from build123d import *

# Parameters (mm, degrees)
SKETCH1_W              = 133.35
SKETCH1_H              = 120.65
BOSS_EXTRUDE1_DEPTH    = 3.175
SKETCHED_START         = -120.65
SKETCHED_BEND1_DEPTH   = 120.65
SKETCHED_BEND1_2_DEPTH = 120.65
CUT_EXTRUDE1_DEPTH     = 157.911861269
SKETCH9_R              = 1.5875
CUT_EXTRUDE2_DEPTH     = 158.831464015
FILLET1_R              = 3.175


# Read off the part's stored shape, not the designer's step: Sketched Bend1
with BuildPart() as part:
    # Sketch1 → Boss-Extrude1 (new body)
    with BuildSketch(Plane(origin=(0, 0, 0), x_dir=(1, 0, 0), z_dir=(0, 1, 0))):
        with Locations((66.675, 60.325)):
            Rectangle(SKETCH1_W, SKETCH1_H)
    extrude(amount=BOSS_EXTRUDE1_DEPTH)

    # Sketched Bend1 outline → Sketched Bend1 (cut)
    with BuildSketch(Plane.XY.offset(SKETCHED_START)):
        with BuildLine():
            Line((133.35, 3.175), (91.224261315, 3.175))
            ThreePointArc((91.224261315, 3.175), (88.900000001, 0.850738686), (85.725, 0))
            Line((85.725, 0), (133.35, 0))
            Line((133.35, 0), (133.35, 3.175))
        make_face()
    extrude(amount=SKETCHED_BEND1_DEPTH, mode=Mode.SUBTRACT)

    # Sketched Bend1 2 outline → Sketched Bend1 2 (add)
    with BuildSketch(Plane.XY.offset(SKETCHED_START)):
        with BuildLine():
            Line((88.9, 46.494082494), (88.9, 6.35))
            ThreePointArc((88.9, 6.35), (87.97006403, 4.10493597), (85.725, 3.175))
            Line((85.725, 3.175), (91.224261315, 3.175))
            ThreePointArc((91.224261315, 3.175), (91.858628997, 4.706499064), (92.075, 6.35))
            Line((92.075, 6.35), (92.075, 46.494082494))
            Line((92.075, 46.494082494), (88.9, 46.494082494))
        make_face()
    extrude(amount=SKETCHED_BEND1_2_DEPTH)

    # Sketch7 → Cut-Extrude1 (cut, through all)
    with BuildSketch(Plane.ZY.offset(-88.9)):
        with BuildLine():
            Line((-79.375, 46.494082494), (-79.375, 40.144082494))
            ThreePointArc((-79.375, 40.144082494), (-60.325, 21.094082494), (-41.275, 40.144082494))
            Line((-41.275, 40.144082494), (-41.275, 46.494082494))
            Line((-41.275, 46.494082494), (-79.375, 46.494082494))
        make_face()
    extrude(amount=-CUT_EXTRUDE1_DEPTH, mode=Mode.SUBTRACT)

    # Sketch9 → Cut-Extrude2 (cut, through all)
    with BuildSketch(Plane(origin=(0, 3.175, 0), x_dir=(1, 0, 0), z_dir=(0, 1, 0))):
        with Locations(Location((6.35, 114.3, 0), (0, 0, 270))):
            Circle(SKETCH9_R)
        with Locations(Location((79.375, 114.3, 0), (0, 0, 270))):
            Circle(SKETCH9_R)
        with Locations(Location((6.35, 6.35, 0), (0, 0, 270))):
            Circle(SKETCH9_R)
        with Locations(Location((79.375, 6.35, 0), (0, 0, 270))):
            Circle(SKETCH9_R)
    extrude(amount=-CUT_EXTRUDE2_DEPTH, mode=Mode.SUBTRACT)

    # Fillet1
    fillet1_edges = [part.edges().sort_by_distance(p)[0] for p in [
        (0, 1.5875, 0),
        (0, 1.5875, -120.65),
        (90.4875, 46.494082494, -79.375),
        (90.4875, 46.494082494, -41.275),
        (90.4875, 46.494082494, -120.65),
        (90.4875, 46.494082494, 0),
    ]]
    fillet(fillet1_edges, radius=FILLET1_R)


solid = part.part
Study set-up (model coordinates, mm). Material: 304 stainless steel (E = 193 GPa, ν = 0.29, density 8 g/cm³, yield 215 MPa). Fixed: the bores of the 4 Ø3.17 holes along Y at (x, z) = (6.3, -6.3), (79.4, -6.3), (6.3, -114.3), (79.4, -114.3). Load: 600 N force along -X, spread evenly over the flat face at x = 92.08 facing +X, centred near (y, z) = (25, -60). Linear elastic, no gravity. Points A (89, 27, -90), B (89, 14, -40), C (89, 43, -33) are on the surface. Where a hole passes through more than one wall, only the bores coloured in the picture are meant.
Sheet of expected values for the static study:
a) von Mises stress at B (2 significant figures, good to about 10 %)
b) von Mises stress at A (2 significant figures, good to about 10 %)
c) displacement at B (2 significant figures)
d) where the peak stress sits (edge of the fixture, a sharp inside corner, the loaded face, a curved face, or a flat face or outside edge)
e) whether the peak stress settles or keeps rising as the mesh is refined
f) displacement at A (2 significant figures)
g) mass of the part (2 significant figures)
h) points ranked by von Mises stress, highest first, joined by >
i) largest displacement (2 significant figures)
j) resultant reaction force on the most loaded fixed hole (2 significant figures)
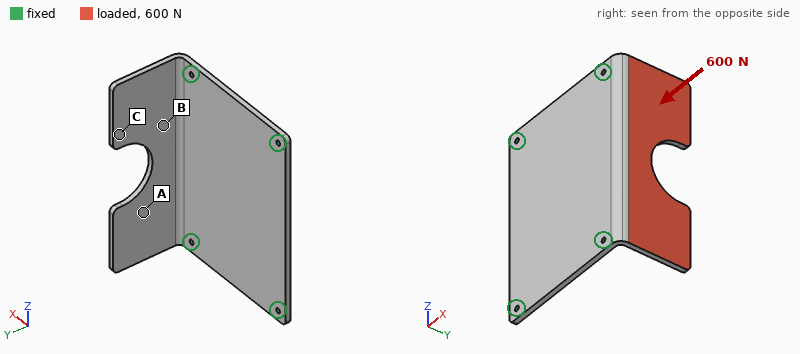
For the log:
32 MPa
18 MPa
0.059 mm
edge of the fixture
keeps rising
0.14 mm
390 g
B > A > C
0.28 mm
220 N
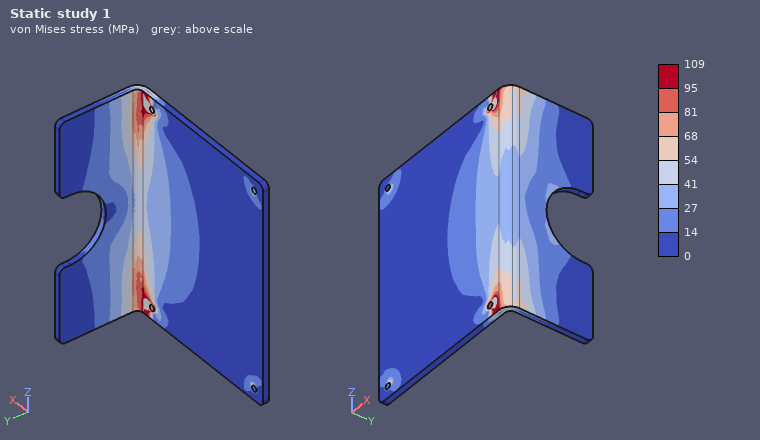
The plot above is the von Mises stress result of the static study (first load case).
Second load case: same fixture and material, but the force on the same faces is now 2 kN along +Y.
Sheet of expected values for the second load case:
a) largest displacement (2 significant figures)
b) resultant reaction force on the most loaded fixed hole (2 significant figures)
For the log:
0.27 mm
1.3 kN
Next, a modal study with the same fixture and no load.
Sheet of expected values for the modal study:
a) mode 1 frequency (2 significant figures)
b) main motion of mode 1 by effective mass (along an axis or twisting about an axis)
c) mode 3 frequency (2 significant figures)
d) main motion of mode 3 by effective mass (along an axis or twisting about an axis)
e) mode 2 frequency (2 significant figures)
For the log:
890 Hz
along X
1300 Hz
along Y
1100 Hz
